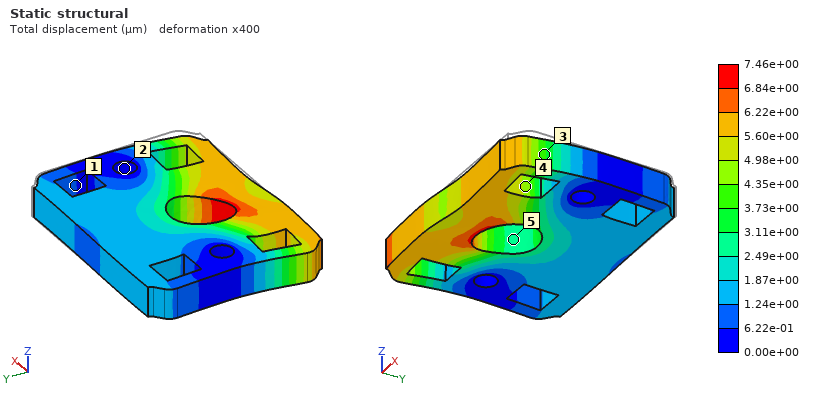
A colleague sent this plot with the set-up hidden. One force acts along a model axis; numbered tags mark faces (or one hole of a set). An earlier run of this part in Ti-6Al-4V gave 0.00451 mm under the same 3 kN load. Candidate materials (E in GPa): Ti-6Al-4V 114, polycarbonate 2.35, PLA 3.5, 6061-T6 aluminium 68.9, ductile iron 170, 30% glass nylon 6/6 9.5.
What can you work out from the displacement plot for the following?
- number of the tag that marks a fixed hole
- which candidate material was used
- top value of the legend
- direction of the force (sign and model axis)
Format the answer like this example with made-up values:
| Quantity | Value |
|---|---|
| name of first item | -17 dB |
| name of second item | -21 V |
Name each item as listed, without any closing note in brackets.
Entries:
| Quantity | Value |
|---|---|
| number of the tag that marks a fixed hole | 2 |
| which candidate material was used | 6061-T6 aluminium |
| top value of the legend | 7.46e+00 µm |
| direction of the force | -X |
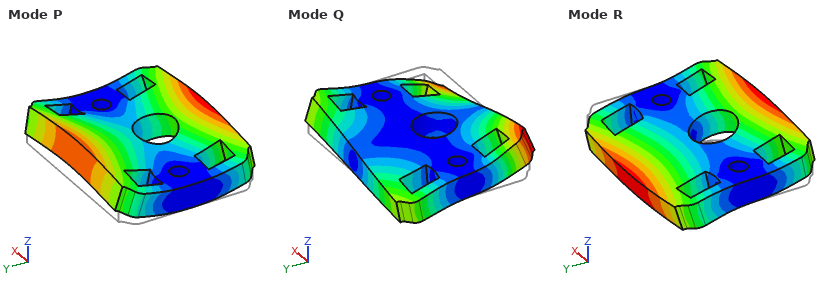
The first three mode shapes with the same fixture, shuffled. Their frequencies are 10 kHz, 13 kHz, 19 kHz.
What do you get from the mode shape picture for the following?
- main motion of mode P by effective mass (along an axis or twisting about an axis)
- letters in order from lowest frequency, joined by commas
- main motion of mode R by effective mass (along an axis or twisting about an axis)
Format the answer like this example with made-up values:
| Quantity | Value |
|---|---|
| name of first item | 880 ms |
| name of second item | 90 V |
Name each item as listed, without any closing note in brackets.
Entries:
| Quantity | Value |
|---|---|
| main motion of mode P by effective mass | along Z |
| letters in order from lowest frequency, joined by commas | R, P, Q |
| main motion of mode R by effective mass | twisting about X |
